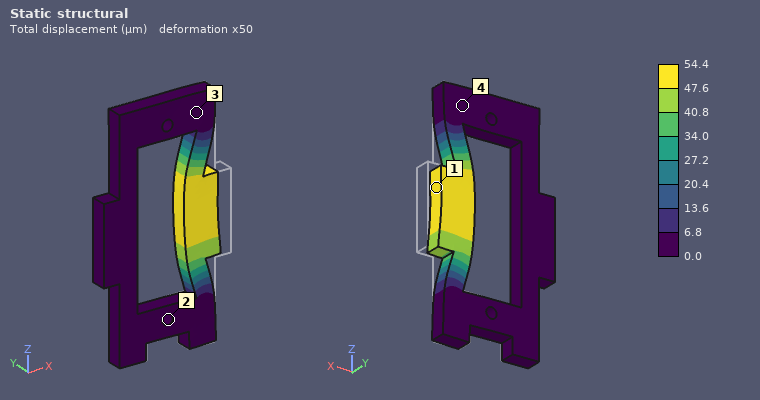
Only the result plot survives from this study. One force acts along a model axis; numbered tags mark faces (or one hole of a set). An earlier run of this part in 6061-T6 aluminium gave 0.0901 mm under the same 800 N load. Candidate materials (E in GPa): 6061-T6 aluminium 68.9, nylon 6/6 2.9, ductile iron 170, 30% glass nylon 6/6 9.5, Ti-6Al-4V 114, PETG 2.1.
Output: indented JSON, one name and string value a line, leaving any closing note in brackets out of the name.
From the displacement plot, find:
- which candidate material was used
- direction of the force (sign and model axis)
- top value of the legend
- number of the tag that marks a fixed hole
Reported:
{
  "which candidate material was used": "Ti-6Al-4V",
  "direction of the force": "-X",
  "top value of the legend": "54.4 µm",
  "number of the tag that marks a fixed hole": "2"
}
